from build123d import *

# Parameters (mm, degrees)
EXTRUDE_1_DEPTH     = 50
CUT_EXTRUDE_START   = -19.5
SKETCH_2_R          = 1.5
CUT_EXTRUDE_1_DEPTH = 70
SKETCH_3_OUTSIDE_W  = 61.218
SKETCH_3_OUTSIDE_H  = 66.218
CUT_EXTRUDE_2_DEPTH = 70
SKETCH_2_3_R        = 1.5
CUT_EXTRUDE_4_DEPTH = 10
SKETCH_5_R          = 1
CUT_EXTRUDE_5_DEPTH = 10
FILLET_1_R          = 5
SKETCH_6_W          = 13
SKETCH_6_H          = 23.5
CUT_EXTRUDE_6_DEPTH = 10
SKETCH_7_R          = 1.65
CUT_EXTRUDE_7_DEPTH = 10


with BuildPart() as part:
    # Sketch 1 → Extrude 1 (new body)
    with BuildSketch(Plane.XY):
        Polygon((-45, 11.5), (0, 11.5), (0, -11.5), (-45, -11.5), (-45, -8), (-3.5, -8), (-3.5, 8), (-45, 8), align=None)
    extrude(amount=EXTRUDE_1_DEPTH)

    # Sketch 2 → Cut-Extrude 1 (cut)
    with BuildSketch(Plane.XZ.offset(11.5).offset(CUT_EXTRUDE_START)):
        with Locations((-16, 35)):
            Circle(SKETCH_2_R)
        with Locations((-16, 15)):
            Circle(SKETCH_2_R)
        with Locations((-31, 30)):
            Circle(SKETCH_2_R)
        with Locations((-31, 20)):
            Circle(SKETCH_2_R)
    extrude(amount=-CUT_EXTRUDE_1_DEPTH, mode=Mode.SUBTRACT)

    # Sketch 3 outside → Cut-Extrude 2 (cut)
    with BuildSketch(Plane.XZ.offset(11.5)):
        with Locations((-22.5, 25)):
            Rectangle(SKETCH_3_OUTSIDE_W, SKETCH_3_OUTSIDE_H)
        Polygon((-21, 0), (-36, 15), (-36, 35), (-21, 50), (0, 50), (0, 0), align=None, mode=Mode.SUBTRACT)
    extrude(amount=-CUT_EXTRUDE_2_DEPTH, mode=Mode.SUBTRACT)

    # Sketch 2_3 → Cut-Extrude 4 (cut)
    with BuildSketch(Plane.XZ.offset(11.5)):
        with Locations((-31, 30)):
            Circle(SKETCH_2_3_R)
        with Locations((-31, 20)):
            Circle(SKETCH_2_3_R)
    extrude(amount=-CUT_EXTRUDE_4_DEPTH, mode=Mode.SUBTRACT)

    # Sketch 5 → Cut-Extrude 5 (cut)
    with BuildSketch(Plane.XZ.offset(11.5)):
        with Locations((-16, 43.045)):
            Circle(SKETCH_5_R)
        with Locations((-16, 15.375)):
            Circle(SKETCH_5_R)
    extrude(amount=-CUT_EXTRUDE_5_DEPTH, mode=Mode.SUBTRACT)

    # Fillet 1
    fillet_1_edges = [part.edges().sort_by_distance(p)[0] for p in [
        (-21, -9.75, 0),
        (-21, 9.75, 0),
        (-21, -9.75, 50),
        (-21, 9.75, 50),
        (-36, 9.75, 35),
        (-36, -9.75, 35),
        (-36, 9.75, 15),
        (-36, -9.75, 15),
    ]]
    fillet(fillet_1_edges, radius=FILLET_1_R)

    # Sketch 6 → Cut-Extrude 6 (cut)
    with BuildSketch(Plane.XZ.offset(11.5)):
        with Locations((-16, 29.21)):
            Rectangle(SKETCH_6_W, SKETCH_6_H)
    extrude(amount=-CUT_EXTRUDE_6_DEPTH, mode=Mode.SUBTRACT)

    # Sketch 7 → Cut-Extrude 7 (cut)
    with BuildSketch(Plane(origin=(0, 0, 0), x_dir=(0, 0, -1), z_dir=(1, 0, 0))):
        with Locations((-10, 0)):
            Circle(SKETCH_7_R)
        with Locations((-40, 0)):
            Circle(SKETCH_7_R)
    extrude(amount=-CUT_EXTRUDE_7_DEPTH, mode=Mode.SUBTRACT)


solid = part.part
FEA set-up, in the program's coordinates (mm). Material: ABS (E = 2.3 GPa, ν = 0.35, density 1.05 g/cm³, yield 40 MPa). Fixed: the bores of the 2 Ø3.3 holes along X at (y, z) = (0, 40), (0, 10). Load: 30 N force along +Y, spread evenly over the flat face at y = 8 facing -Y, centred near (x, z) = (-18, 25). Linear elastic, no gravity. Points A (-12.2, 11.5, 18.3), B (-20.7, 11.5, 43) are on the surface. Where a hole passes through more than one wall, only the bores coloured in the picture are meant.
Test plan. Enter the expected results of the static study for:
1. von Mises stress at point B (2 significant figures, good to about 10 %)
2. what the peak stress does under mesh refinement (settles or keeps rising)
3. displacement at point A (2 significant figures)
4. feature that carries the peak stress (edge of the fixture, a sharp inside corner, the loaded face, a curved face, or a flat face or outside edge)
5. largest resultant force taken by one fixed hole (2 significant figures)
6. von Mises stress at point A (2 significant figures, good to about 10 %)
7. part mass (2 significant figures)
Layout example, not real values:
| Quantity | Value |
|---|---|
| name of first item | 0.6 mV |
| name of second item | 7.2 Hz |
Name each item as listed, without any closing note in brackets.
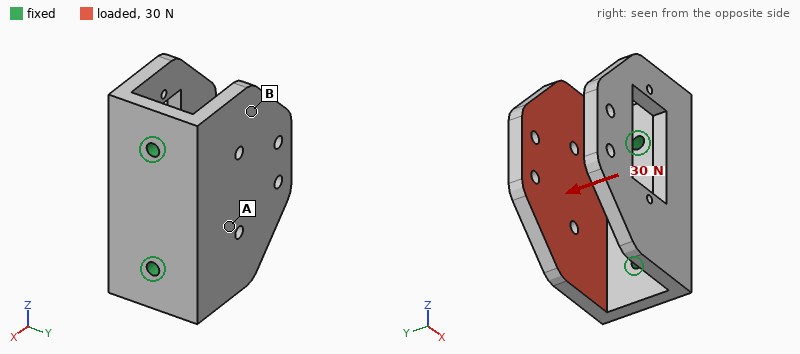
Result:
| Quantity | Value |
|---|---|
| von Mises stress at point B | 0.95 MPa |
| what the peak stress does under mesh refinement | keeps rising |
| displacement at point A | 0.19 mm |
| feature that carries the peak stress | edge of the fixture |
| largest resultant force taken by one fixed hole | 15 N |
| von Mises stress at point A | 1.9 MPa |
| part mass | 13 g |
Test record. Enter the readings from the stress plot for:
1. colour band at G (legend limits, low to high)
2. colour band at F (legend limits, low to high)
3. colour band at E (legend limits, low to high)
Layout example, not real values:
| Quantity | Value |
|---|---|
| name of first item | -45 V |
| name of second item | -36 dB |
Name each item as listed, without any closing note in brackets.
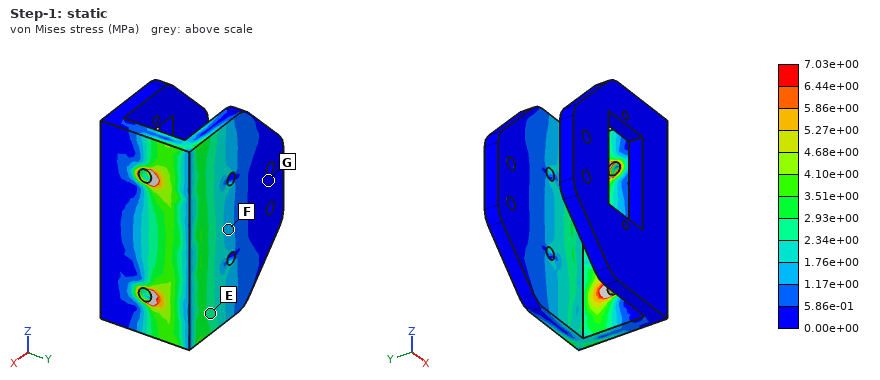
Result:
| Quantity | Value |
|---|---|
| colour band at G | 0.00e+00 to 5.86e-01 MPa |
| colour band at F | 1.17e+00 to 1.76e+00 MPa |
| colour band at E | 2.34e+00 to 2.93e+00 MPa |
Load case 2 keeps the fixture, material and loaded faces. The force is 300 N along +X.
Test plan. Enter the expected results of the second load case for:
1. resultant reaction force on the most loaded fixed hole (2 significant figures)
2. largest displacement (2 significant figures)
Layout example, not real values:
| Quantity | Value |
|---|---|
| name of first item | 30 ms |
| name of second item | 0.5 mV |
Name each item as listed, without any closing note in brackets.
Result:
| Quantity | Value |
|---|---|
| resultant reaction force on the most loaded fixed hole | 150 N |
| largest displacement | 0.63 mm |
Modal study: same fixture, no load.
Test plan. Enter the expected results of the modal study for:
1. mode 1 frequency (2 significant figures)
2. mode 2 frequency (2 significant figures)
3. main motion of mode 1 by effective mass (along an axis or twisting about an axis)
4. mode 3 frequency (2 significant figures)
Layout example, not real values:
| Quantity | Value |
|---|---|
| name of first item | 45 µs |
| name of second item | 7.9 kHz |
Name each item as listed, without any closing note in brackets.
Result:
| Quantity | Value |
|---|---|
| mode 1 frequency | 540 Hz |
| mode 2 frequency | 620 Hz |
| main motion of mode 1 by effective mass | along Y |
| mode 3 frequency | 1300 Hz |
